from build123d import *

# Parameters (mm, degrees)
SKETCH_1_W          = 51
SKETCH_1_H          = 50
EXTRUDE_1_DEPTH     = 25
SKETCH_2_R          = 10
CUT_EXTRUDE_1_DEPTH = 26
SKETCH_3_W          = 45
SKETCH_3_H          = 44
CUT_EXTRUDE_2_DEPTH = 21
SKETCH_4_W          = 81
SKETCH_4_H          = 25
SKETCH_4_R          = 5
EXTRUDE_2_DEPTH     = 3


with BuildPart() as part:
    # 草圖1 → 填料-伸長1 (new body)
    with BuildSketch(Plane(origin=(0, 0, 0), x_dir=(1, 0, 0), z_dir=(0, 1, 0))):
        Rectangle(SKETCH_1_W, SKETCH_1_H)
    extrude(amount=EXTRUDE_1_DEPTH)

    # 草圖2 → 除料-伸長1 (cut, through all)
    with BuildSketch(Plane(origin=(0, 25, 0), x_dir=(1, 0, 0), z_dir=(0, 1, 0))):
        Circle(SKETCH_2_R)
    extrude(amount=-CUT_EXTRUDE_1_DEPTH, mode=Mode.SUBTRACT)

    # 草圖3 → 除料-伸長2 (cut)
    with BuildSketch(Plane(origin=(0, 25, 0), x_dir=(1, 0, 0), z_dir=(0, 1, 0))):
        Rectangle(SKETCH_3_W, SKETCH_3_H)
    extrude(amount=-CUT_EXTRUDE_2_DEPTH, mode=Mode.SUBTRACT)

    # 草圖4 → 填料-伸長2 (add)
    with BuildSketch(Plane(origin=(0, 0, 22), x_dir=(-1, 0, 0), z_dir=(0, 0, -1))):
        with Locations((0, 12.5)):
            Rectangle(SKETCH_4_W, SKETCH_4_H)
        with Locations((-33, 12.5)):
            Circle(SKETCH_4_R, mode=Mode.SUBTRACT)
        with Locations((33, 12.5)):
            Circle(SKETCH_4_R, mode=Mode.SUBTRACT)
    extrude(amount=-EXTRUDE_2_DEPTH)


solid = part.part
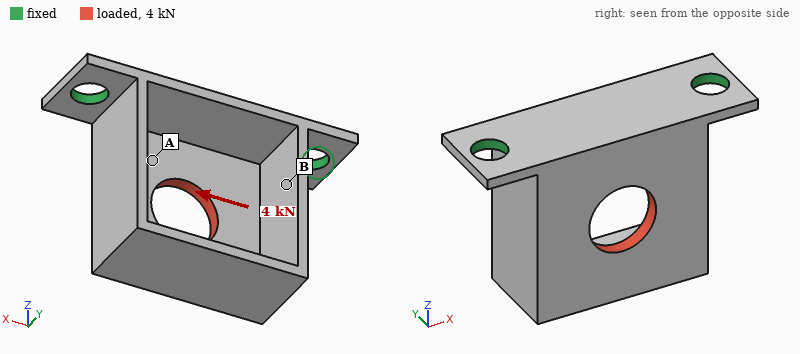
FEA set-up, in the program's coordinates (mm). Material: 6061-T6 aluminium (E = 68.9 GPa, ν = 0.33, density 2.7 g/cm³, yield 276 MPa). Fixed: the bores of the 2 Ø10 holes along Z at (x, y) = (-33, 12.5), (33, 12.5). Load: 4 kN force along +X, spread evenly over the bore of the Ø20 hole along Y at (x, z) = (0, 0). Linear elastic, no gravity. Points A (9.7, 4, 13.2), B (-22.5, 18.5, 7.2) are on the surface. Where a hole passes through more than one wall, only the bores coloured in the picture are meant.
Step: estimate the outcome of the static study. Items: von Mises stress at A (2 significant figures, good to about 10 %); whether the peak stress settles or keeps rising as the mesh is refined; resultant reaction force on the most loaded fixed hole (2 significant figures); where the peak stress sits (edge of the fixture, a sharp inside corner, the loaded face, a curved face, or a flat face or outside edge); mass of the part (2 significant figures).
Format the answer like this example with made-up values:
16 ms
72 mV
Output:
52 MPa
keeps rising
2.7 kN
edge of the fixture
61 g
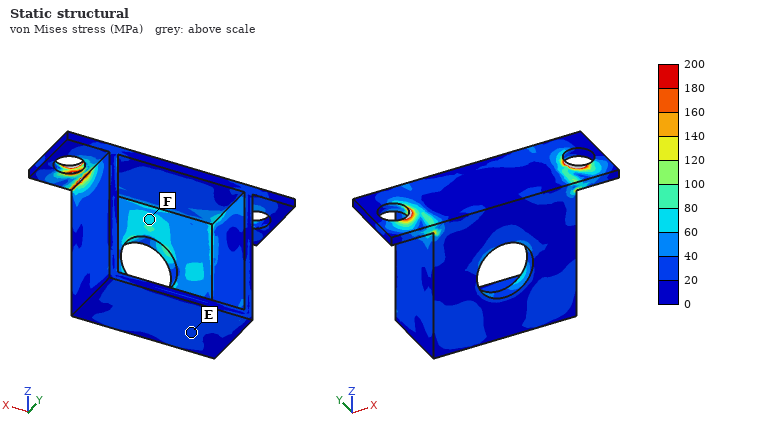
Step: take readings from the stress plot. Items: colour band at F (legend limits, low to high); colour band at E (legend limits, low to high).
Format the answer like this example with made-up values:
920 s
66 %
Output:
60 to 80 MPa
20 to 40 MPa
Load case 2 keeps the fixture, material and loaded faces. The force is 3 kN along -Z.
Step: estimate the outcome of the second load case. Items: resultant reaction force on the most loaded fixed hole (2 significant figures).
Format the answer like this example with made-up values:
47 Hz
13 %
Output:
1.6 kN
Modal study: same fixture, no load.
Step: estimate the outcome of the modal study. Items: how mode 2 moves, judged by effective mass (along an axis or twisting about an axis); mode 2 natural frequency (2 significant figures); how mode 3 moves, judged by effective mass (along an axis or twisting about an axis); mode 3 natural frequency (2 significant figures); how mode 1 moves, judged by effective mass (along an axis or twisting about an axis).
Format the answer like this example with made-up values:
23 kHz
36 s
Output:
along X
2000 Hz
along Z
6400 Hz
along Y
